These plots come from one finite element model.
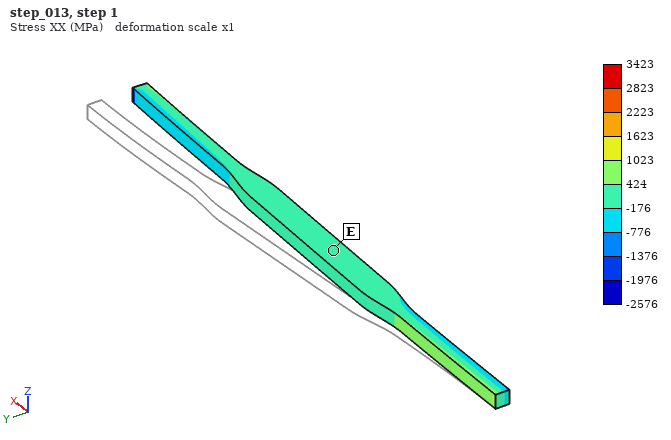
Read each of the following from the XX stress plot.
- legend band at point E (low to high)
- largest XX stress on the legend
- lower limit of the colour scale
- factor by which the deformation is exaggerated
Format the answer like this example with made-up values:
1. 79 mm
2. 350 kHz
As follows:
1. -176 to 424 MPa
2. 3423 MPa
3. -2576 MPa
4. 1
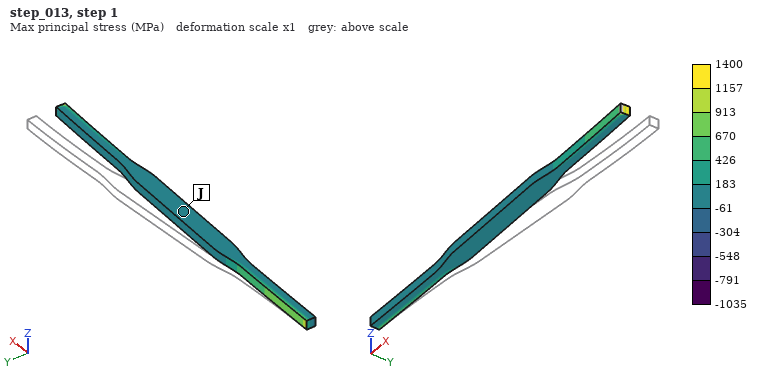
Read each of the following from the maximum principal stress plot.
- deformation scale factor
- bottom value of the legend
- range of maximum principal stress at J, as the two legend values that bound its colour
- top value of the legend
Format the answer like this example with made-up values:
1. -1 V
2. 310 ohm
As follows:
1. 1
2. -1035 MPa
3. -61 to 183 MPa
4. 1400 MPa
